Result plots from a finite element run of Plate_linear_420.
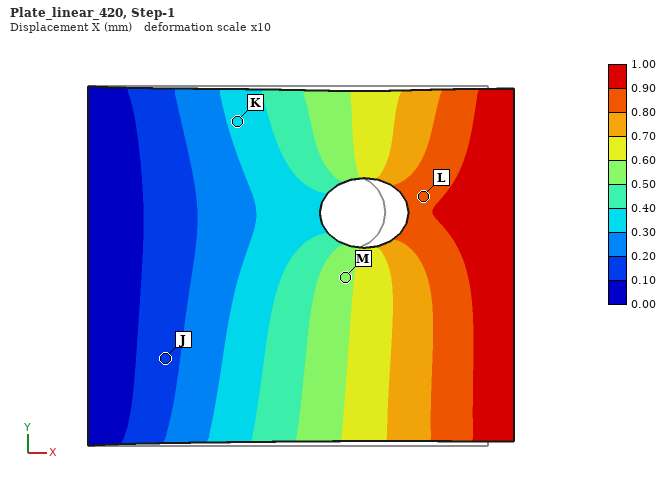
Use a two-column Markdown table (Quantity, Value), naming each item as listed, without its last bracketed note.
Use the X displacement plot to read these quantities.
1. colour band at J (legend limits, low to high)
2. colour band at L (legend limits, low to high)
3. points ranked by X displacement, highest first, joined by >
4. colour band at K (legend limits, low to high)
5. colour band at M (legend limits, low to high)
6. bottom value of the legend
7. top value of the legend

| Quantity | Value |
|---|---|
| colour band at J | 0.10 to 0.20 mm |
| colour band at L | 0.80 to 0.90 mm |
| points ranked by X displacement, highest first, joined by > | L > M > K > J |
| colour band at K | 0.30 to 0.40 mm |
| colour band at M | 0.50 to 0.60 mm |
| bottom value of the legend | 0.00 mm |
| top value of the legend | 1.00 mm |
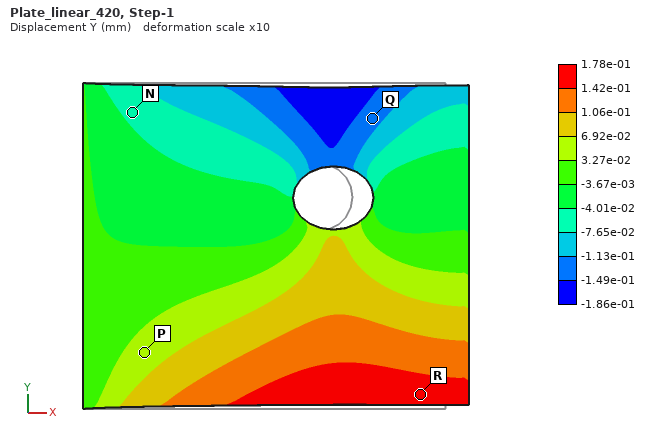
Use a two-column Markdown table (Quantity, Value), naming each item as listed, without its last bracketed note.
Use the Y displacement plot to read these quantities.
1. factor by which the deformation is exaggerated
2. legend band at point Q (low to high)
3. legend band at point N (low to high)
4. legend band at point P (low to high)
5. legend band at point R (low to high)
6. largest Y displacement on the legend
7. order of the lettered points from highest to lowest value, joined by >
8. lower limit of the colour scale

| Quantity | Value |
|---|---|
| factor by which the deformation is exaggerated | 10 |
| legend band at point Q | -1.49e-01 to -1.13e-01 mm |
| legend band at point N | -7.65e-02 to -4.01e-02 mm |
| legend band at point P | 3.27e-02 to 6.92e-02 mm |
| legend band at point R | 1.42e-01 to 1.78e-01 mm |
| largest Y displacement on the legend | 1.78e-01 mm |
| order of the lettered points from highest to lowest value, joined by > | R > P > N > Q |
| lower limit of the colour scale | -1.86e-01 mm |
